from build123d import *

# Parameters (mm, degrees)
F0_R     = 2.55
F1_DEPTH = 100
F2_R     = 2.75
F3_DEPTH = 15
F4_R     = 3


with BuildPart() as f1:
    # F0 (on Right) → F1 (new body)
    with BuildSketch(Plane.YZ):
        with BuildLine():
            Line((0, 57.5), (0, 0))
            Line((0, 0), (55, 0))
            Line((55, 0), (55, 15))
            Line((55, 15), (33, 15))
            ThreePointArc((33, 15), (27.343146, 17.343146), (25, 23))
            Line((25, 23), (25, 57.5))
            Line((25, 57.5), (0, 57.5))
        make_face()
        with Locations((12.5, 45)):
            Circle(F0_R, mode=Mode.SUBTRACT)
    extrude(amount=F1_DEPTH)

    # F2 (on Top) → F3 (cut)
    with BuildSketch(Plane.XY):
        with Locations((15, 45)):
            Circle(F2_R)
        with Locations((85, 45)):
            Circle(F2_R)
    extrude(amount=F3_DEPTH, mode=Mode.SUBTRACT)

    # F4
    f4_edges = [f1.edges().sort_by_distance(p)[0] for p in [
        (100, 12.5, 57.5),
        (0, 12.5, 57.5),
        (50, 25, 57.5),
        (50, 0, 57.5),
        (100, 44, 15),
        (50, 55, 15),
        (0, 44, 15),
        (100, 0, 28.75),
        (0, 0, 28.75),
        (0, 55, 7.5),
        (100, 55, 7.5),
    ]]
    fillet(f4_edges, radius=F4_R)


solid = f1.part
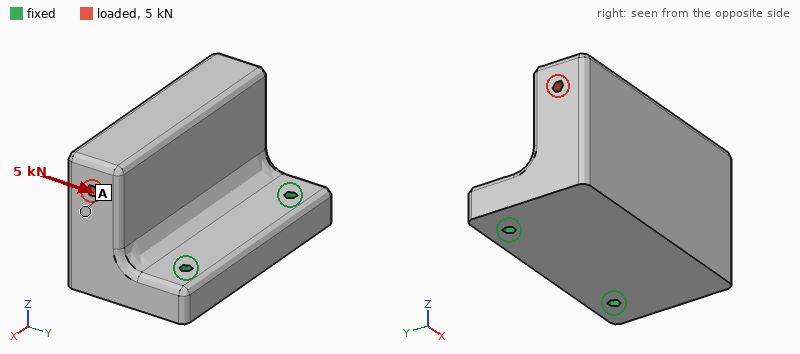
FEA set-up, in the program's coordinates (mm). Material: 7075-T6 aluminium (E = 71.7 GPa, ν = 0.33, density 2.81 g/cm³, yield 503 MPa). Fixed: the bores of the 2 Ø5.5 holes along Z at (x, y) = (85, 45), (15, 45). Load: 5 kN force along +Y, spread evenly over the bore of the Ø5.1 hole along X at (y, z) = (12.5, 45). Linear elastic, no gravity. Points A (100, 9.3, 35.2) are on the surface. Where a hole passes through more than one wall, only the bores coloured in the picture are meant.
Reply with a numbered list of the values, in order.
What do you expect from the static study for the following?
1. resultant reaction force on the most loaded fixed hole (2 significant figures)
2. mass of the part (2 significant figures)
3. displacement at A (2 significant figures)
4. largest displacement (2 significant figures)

1. 2.6 kN
2. 520 g
3. 0.12 mm
4. 0.20 mm
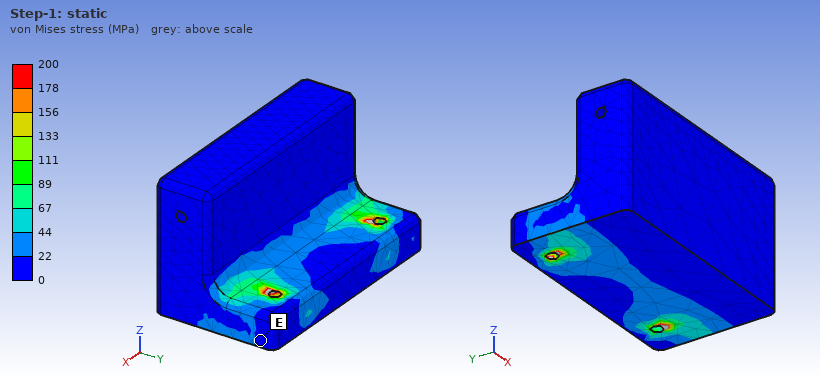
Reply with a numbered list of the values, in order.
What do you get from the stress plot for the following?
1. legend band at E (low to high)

1. 0 to 22 MPa
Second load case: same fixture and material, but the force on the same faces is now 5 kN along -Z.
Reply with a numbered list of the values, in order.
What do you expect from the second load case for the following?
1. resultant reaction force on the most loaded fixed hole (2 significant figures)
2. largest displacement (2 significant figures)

1. 2.5 kN
2. 0.13 mm
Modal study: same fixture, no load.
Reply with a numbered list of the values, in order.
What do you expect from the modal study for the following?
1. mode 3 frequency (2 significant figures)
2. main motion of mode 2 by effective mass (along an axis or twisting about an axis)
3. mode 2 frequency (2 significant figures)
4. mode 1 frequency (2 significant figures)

1. 6500 Hz
2. along X
3. 4000 Hz
4. 1600 Hz
